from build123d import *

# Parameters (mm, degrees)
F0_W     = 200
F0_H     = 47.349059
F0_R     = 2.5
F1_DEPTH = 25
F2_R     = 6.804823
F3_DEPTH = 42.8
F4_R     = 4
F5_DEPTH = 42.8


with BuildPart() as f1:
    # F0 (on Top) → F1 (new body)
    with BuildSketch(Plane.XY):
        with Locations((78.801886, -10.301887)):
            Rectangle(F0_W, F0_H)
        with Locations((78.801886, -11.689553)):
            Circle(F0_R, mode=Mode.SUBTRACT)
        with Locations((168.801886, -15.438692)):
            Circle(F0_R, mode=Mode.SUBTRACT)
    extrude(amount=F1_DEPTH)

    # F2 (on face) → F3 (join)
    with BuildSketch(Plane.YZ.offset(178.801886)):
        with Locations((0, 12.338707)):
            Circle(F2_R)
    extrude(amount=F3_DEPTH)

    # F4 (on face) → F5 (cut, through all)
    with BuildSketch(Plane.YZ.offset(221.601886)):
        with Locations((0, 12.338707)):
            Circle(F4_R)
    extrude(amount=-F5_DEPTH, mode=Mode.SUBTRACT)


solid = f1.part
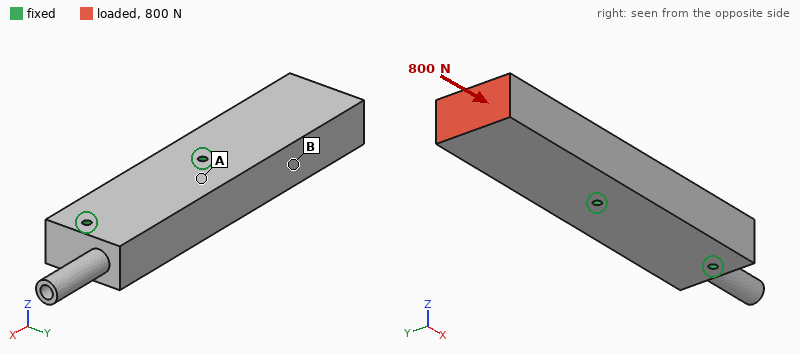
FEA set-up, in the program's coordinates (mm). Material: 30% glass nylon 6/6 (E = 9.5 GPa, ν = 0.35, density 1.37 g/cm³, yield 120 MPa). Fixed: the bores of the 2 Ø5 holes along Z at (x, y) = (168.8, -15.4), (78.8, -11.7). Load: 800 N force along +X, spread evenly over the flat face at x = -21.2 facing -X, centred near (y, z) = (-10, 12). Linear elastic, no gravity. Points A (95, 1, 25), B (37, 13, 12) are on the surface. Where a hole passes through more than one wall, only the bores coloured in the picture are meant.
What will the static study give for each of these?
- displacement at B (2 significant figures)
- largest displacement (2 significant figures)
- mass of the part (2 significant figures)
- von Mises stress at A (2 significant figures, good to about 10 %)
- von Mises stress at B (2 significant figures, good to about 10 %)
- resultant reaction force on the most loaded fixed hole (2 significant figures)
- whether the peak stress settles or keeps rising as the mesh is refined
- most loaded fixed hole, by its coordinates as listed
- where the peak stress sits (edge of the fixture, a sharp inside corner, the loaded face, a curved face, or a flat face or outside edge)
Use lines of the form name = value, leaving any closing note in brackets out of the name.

displacement at B = 4.7 µm
largest displacement = 8.9 µm
mass of the part = 330 g
von Mises stress at A = 0.27 MPa
von Mises stress at B = 0.67 MPa
resultant reaction force on the most loaded fixed hole = 690 N
whether the peak stress settles or keeps rising as the mesh is refined = keeps rising
most loaded fixed hole, by its coordinates as listed = (78.8, -11.7)
where the peak stress sits = edge of the fixture
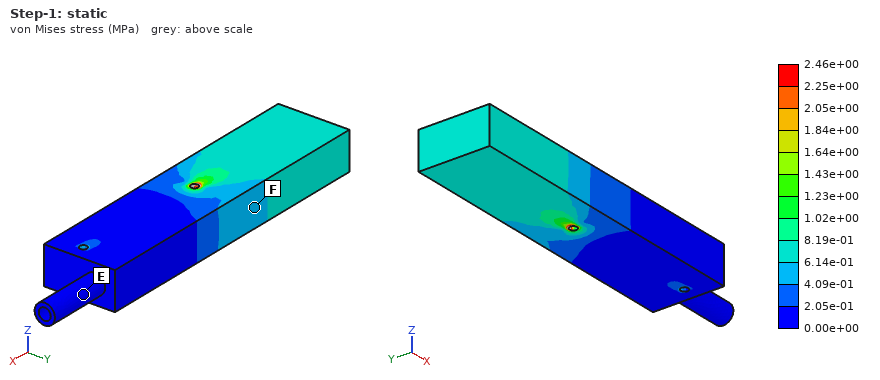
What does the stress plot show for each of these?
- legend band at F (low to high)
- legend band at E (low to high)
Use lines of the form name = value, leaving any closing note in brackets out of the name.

legend band at F = 4.09e-01 to 6.14e-01 MPa
legend band at E = 0.00e+00 to 2.05e-01 MPa
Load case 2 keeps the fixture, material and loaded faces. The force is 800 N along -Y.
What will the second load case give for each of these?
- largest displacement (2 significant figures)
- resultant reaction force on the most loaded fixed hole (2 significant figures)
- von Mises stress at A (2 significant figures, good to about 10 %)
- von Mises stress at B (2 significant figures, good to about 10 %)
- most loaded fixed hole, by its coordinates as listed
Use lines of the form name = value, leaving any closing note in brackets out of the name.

largest displacement = 0.29 mm
resultant reaction force on the most loaded fixed hole = 1.6 kN
von Mises stress at A = 3.2 MPa
von Mises stress at B = 5.0 MPa
most loaded fixed hole, by its coordinates as listed = (78.8, -11.7)
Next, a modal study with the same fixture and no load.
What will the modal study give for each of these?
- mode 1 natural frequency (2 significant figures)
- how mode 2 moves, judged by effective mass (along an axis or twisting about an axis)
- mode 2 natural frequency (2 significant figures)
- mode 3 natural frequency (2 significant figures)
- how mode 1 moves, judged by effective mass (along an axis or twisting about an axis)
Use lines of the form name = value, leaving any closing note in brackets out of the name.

mode 1 natural frequency = 890 Hz
how mode 2 moves, judged by effective mass = along Y
mode 2 natural frequency = 1200 Hz
mode 3 natural frequency = 2500 Hz
how mode 1 moves, judged by effective mass = along Z
